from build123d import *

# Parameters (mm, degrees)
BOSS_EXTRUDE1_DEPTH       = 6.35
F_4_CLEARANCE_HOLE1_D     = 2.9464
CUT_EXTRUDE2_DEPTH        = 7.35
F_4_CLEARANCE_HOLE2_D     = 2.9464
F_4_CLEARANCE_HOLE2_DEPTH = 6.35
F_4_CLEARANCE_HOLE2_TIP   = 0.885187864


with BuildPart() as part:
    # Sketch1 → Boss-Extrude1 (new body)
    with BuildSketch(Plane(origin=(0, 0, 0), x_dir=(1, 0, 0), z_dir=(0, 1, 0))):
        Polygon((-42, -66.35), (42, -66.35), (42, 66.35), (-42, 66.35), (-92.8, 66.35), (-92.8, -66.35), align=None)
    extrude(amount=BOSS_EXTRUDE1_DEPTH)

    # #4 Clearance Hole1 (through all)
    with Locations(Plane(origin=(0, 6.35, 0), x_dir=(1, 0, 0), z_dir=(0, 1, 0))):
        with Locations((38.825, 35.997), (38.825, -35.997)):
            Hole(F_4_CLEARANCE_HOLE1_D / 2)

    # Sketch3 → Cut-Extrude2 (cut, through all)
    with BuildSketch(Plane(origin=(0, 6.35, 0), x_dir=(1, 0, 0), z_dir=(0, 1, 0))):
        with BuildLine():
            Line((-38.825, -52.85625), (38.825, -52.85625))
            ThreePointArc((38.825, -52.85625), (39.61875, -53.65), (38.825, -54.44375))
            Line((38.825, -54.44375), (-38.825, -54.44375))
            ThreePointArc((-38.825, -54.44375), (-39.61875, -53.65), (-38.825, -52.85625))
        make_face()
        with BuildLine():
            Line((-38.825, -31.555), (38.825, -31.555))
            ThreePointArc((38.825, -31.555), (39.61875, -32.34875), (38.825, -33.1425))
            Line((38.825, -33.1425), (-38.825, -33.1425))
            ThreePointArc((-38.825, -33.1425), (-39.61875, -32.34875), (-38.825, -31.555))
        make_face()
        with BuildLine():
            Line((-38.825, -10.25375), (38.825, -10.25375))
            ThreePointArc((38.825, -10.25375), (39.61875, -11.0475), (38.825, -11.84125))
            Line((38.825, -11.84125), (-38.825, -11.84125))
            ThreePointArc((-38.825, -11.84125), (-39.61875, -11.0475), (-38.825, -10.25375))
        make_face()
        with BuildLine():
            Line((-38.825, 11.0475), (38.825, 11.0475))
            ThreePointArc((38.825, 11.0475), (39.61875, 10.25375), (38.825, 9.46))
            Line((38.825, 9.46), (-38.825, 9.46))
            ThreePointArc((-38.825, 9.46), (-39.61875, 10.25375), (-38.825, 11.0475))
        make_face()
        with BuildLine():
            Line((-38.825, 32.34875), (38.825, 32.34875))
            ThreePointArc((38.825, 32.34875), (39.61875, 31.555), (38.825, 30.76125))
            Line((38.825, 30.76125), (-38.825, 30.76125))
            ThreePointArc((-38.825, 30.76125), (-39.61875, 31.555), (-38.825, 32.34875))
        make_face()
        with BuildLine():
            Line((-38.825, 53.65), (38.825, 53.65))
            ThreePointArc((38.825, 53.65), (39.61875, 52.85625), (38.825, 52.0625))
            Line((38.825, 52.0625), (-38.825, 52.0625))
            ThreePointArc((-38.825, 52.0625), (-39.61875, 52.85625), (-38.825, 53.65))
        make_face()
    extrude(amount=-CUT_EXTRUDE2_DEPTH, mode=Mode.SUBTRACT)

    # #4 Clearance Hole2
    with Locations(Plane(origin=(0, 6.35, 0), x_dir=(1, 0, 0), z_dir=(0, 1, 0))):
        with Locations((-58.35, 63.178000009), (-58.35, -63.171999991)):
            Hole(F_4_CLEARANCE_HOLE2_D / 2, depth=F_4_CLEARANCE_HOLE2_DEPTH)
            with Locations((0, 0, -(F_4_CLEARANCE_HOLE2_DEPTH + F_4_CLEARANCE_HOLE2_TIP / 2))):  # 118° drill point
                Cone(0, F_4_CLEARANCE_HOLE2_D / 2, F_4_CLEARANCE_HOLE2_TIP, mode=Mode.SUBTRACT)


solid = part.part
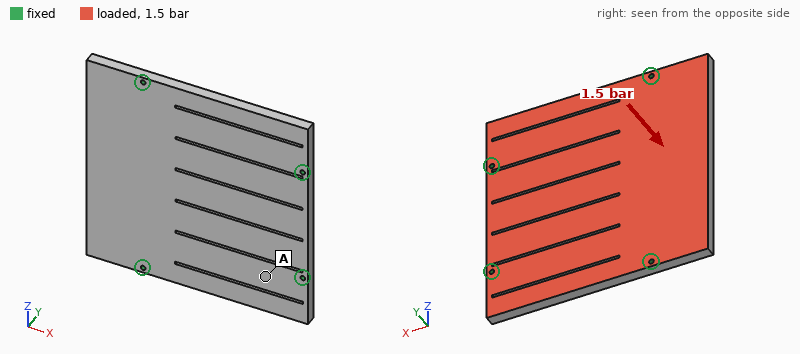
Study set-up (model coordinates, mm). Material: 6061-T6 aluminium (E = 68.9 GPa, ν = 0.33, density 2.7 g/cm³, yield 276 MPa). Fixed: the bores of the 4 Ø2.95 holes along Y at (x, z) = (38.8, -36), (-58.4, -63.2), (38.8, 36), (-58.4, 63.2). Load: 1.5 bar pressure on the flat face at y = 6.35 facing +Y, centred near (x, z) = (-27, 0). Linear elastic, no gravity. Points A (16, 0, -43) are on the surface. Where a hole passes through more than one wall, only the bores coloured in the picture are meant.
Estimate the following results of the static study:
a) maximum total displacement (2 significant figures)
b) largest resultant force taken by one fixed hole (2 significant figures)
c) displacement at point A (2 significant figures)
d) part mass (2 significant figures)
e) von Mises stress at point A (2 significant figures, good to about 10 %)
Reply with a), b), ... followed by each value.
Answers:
a) 0.19 mm
b) 830 N
c) 0.030 mm
d) 290 g
e) 13 MPa
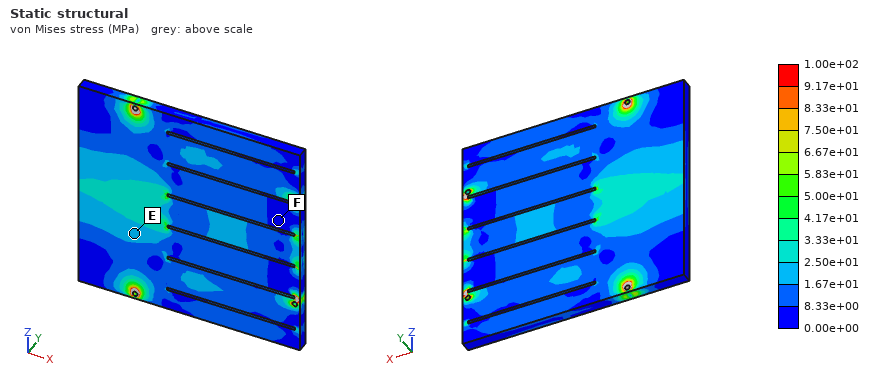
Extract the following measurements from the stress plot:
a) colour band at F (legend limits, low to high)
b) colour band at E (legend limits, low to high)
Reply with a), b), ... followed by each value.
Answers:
a) 0.00e+00 to 8.33e+00 MPa
b) 1.67e+01 to 2.50e+01 MPa
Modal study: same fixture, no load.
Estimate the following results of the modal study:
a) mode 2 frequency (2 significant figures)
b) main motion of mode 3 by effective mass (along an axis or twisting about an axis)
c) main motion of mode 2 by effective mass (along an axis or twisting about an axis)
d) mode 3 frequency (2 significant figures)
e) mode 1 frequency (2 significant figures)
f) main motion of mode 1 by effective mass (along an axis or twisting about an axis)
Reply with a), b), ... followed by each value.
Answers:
a) 1700 Hz
b) twisting about X
c) twisting about Z
d) 2300 Hz
e) 1300 Hz
f) along Y
